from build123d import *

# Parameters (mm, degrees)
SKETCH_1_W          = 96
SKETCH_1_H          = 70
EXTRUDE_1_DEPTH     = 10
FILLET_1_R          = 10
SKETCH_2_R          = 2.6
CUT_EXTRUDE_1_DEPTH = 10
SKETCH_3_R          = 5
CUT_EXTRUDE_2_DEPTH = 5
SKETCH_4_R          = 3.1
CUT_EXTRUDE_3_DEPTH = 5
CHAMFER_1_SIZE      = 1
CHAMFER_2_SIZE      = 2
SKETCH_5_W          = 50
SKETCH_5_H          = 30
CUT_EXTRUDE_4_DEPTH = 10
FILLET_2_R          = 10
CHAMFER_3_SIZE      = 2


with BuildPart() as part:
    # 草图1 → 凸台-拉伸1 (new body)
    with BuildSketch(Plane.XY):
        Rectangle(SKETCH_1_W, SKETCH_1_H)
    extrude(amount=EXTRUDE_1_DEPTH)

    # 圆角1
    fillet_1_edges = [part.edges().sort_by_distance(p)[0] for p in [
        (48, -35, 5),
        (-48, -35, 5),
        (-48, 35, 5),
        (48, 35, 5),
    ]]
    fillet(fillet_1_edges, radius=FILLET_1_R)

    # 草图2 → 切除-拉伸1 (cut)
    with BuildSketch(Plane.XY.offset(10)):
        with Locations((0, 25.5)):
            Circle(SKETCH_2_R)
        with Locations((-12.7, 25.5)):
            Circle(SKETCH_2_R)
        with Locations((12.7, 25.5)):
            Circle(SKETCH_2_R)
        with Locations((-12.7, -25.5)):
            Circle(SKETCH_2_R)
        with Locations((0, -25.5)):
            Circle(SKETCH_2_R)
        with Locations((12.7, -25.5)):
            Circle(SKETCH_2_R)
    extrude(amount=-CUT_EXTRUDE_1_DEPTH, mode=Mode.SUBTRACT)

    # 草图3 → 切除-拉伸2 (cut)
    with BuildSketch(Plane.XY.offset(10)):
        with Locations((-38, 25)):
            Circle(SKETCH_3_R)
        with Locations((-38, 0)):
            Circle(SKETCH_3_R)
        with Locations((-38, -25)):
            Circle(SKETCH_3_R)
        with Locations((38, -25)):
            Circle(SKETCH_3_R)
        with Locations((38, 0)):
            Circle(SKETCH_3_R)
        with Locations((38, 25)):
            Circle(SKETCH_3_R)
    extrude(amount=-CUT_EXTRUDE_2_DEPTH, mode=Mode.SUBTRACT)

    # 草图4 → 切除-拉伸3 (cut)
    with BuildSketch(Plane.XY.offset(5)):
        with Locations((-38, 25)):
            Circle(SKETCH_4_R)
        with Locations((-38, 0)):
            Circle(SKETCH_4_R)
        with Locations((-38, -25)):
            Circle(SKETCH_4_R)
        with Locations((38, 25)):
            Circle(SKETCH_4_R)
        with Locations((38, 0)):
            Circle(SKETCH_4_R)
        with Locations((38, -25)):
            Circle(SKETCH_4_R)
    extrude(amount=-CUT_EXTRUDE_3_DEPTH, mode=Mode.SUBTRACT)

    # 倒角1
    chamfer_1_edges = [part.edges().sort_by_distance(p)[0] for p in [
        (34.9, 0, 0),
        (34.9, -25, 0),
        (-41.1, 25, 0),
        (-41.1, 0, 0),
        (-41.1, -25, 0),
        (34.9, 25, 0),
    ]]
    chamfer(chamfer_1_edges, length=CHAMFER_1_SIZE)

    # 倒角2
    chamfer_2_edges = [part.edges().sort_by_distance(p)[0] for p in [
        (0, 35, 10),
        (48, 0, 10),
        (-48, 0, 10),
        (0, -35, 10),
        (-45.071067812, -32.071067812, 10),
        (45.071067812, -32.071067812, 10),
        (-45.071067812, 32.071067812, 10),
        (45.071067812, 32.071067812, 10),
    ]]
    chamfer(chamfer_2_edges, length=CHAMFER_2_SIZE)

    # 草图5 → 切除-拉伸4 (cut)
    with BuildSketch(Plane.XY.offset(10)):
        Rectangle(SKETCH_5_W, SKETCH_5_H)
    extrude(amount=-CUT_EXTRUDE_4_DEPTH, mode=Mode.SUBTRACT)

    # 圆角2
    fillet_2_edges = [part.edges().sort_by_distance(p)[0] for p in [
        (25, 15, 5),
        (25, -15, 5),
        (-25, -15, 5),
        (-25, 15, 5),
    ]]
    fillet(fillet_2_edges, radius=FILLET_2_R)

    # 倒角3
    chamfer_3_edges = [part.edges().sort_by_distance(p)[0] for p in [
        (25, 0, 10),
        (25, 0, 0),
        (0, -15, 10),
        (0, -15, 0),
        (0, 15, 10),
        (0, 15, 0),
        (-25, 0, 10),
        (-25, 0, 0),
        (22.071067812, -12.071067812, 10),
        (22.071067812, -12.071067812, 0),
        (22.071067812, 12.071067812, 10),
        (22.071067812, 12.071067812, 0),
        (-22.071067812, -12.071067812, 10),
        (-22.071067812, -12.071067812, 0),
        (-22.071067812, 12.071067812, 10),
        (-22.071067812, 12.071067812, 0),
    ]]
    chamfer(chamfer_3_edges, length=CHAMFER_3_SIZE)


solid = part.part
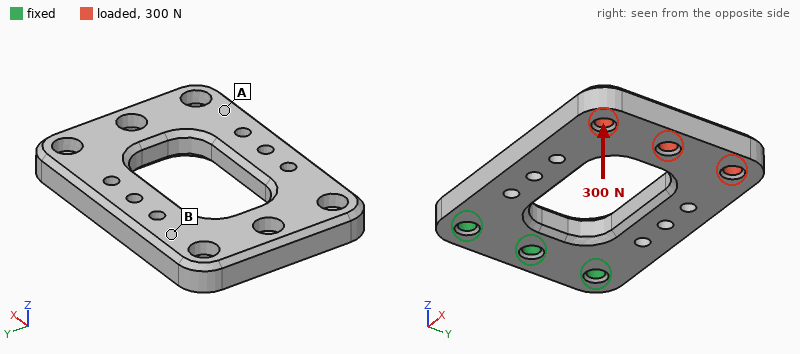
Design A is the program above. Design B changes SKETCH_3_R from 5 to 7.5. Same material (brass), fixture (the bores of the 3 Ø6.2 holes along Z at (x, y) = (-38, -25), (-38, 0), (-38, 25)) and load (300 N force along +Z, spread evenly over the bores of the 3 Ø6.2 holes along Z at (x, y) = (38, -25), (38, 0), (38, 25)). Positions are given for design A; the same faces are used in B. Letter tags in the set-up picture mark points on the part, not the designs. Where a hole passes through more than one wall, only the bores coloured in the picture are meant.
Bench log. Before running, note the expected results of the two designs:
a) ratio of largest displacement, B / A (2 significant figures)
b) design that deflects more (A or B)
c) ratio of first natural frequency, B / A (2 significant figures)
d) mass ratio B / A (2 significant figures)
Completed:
1.1
B
0.99
0.94
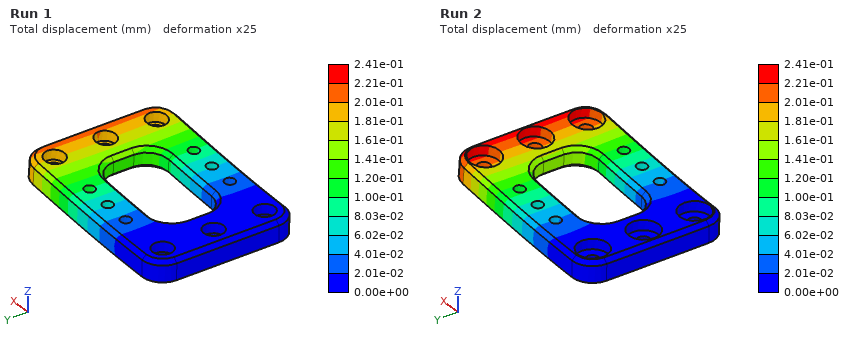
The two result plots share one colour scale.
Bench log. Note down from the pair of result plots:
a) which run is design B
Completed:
Run 2
